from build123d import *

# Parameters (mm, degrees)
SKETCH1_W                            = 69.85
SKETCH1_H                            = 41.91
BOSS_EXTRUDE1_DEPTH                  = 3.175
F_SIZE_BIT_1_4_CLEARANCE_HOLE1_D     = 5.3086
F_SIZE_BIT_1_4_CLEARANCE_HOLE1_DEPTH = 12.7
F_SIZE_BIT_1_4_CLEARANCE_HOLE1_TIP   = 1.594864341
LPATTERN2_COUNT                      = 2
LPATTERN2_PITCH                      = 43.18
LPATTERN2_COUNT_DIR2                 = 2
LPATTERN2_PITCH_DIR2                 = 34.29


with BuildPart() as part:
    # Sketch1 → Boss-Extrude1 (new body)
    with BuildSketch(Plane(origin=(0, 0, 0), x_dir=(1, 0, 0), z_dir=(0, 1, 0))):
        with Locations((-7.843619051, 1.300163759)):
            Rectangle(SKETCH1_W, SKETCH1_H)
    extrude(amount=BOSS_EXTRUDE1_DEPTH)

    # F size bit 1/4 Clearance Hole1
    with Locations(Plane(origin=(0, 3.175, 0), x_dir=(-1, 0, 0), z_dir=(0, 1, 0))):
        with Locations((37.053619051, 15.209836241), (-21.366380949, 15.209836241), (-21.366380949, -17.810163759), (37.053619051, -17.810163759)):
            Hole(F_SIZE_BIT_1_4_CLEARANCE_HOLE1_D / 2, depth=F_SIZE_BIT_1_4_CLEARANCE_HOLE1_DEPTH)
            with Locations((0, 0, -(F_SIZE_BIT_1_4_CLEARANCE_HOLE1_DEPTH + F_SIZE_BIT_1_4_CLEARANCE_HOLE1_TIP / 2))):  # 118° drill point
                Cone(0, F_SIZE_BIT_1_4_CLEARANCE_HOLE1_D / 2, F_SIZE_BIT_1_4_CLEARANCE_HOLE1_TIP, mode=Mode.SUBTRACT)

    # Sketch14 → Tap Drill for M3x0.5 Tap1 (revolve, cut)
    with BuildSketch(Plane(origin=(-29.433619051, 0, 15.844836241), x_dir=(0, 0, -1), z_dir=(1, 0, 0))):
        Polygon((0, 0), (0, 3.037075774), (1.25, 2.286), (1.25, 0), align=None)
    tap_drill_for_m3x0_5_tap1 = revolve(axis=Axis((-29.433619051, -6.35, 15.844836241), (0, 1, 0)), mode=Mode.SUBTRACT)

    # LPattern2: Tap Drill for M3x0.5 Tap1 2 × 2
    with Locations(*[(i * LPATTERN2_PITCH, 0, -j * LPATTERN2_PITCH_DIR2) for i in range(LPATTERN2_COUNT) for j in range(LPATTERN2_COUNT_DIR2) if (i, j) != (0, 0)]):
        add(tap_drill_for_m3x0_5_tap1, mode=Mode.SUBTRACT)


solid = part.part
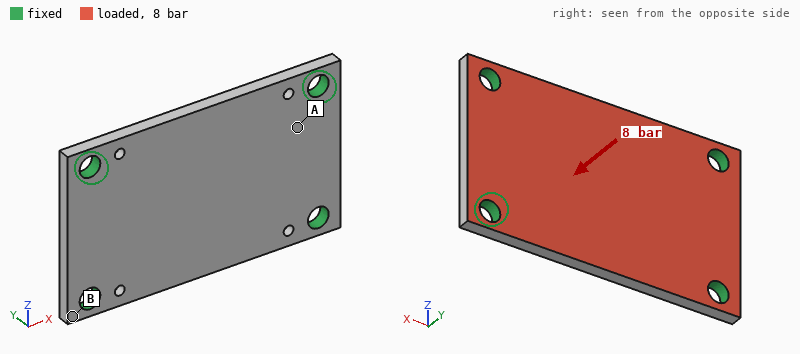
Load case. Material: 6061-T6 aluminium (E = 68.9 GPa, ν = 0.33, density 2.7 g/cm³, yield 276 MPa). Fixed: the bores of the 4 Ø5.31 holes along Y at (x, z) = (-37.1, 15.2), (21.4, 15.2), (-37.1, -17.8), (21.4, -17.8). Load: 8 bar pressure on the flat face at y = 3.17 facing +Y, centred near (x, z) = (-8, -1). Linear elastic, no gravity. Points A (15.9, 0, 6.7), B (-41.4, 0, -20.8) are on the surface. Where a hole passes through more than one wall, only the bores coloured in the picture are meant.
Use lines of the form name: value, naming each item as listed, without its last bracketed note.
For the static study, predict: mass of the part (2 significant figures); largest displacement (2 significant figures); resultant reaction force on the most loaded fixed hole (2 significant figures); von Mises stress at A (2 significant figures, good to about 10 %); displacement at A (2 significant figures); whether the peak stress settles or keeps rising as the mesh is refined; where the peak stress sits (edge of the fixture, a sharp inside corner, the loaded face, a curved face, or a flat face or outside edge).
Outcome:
mass of the part: 24 g
largest displacement: 0.14 mm
resultant reaction force on the most loaded fixed hole: 570 N
von Mises stress at A: 43 MPa
displacement at A: 0.030 mm
whether the peak stress settles or keeps rising as the mesh is refined: keeps rising
where the peak stress sits: edge of the fixture
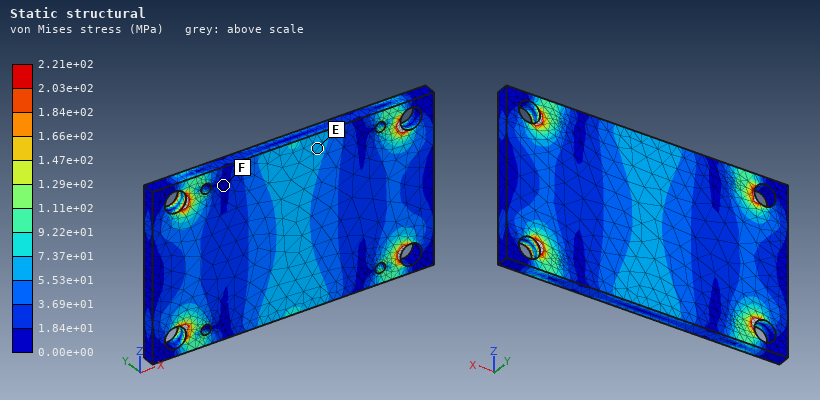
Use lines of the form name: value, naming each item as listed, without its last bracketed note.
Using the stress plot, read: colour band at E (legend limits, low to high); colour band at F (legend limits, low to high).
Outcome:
colour band at E: 5.53e+01 to 7.37e+01 MPa
colour band at F: 0.00e+00 to 1.84e+01 MPa
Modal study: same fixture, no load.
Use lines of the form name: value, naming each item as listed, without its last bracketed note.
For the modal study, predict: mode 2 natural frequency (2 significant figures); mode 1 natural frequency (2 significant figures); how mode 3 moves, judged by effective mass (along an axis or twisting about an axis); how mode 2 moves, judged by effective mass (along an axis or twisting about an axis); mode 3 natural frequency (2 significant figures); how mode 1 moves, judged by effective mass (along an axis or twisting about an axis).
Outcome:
mode 2 natural frequency: 7000 Hz
mode 1 natural frequency: 4700 Hz
how mode 3 moves, judged by effective mass: twisting about Z
how mode 2 moves, judged by effective mass: twisting about X
mode 3 natural frequency: 12 kHz
how mode 1 moves, judged by effective mass: along Y
